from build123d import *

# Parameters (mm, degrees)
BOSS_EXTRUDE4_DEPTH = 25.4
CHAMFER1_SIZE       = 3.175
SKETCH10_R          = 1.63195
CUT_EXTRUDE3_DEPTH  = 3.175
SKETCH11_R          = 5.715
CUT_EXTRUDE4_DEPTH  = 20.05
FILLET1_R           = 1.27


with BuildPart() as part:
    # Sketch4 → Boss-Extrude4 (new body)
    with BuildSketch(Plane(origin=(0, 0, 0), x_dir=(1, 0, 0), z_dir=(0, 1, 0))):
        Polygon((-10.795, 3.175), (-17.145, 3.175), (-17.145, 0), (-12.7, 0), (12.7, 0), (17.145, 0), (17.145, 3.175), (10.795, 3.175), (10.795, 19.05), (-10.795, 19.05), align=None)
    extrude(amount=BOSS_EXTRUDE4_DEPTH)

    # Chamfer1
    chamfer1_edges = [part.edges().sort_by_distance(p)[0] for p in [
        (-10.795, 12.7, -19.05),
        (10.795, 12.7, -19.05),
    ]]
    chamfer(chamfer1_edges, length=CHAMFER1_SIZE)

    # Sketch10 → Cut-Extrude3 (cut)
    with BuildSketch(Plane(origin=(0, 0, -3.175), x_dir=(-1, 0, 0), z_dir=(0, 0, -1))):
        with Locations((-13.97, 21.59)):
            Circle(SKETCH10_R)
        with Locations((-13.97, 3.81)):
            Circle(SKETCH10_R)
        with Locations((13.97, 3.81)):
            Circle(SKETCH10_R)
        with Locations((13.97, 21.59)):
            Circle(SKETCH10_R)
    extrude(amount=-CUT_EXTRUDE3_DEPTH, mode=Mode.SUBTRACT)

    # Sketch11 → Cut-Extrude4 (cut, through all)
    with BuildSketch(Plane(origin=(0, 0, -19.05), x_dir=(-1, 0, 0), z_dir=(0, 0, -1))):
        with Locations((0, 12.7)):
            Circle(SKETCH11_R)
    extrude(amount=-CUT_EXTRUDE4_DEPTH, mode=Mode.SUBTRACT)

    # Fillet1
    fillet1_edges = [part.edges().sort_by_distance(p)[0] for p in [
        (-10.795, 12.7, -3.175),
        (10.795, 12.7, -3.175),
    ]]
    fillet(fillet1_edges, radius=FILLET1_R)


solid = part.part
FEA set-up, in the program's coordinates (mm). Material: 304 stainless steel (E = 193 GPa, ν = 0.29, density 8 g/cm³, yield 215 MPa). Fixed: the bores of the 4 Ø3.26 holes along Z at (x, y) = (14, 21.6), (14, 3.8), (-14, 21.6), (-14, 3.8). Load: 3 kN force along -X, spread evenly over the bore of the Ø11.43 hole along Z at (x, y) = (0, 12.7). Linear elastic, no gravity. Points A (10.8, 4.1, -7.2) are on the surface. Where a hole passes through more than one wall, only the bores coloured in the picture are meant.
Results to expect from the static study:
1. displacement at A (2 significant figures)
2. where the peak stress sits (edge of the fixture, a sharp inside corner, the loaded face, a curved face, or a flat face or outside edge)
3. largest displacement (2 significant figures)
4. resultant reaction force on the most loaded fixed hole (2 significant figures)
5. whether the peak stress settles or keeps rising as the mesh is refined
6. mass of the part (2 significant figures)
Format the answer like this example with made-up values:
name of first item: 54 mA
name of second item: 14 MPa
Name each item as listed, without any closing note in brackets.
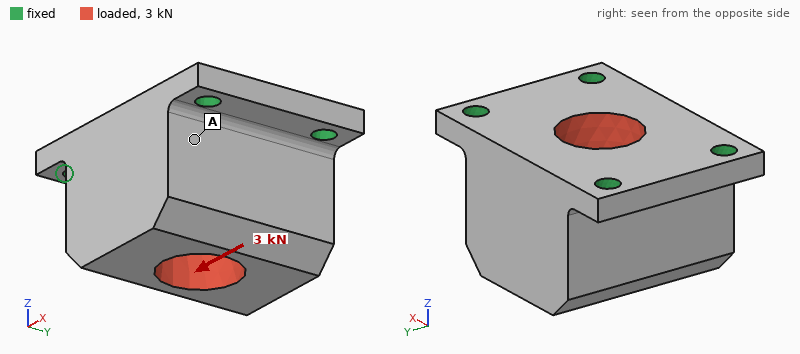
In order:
displacement at A: 1.8 µm
where the peak stress sits: edge of the fixture
largest displacement: 3.8 µm
resultant reaction force on the most loaded fixed hole: 900 N
whether the peak stress settles or keeps rising as the mesh is refined: keeps rising
mass of the part: 73 g
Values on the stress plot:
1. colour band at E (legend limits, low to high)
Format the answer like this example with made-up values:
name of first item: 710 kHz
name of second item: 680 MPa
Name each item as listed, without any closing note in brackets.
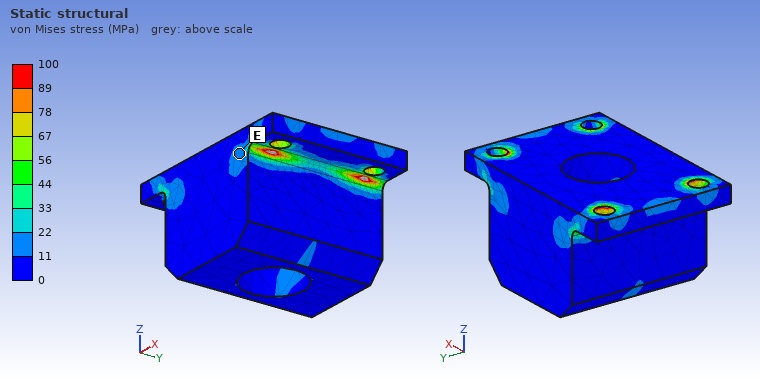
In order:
colour band at E: 11 to 22 MPa
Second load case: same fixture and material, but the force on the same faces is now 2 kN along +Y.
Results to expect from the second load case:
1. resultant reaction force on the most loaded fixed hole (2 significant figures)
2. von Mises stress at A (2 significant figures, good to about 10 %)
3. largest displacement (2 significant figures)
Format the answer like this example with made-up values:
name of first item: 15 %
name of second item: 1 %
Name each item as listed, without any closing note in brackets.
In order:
resultant reaction force on the most loaded fixed hole: 730 N
von Mises stress at A: 13 MPa
largest displacement: 4.9 µm
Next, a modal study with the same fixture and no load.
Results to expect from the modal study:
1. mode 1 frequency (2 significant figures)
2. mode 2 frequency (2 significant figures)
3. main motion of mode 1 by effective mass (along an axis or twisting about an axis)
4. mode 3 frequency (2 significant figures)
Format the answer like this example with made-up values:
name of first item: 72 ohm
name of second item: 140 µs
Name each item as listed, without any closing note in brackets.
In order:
mode 1 frequency: 14 kHz
mode 2 frequency: 21 kHz
main motion of mode 1 by effective mass: along Y
mode 3 frequency: 21 kHz
